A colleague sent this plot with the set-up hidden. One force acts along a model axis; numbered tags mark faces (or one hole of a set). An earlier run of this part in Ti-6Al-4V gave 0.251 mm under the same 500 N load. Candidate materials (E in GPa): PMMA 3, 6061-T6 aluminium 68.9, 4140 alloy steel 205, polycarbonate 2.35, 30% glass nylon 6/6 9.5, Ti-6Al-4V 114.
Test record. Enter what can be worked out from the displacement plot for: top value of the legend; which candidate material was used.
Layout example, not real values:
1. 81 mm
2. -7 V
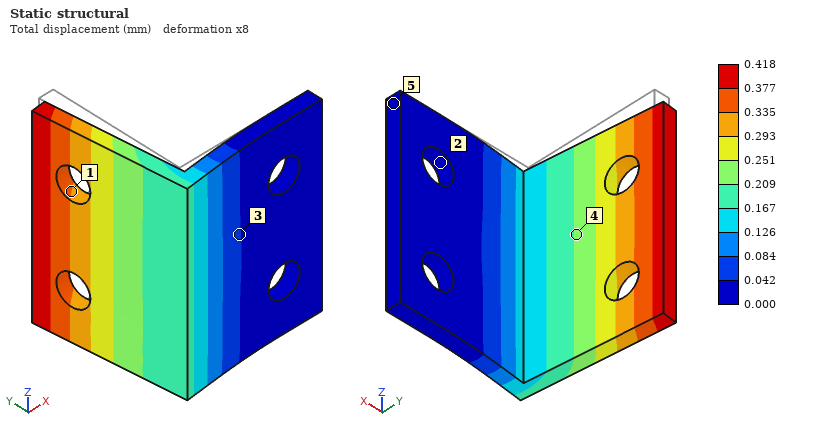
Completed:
1. 0.418 mm
2. 6061-T6 aluminium
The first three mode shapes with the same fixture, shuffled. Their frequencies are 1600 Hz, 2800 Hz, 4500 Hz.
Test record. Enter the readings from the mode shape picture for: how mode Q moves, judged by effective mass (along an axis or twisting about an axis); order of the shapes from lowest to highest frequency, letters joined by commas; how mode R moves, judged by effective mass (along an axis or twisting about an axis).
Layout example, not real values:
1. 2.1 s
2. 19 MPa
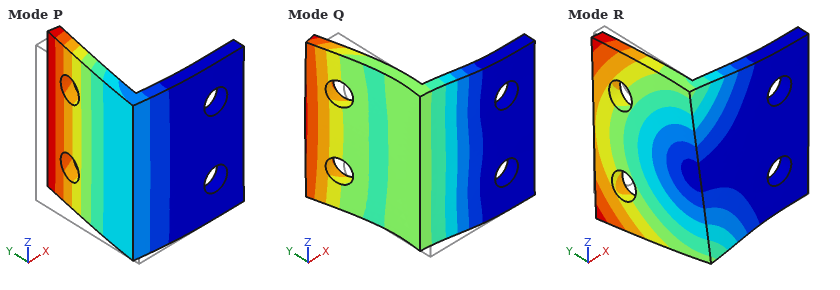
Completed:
1. along Y
2. P, R, Q
3. along Z
